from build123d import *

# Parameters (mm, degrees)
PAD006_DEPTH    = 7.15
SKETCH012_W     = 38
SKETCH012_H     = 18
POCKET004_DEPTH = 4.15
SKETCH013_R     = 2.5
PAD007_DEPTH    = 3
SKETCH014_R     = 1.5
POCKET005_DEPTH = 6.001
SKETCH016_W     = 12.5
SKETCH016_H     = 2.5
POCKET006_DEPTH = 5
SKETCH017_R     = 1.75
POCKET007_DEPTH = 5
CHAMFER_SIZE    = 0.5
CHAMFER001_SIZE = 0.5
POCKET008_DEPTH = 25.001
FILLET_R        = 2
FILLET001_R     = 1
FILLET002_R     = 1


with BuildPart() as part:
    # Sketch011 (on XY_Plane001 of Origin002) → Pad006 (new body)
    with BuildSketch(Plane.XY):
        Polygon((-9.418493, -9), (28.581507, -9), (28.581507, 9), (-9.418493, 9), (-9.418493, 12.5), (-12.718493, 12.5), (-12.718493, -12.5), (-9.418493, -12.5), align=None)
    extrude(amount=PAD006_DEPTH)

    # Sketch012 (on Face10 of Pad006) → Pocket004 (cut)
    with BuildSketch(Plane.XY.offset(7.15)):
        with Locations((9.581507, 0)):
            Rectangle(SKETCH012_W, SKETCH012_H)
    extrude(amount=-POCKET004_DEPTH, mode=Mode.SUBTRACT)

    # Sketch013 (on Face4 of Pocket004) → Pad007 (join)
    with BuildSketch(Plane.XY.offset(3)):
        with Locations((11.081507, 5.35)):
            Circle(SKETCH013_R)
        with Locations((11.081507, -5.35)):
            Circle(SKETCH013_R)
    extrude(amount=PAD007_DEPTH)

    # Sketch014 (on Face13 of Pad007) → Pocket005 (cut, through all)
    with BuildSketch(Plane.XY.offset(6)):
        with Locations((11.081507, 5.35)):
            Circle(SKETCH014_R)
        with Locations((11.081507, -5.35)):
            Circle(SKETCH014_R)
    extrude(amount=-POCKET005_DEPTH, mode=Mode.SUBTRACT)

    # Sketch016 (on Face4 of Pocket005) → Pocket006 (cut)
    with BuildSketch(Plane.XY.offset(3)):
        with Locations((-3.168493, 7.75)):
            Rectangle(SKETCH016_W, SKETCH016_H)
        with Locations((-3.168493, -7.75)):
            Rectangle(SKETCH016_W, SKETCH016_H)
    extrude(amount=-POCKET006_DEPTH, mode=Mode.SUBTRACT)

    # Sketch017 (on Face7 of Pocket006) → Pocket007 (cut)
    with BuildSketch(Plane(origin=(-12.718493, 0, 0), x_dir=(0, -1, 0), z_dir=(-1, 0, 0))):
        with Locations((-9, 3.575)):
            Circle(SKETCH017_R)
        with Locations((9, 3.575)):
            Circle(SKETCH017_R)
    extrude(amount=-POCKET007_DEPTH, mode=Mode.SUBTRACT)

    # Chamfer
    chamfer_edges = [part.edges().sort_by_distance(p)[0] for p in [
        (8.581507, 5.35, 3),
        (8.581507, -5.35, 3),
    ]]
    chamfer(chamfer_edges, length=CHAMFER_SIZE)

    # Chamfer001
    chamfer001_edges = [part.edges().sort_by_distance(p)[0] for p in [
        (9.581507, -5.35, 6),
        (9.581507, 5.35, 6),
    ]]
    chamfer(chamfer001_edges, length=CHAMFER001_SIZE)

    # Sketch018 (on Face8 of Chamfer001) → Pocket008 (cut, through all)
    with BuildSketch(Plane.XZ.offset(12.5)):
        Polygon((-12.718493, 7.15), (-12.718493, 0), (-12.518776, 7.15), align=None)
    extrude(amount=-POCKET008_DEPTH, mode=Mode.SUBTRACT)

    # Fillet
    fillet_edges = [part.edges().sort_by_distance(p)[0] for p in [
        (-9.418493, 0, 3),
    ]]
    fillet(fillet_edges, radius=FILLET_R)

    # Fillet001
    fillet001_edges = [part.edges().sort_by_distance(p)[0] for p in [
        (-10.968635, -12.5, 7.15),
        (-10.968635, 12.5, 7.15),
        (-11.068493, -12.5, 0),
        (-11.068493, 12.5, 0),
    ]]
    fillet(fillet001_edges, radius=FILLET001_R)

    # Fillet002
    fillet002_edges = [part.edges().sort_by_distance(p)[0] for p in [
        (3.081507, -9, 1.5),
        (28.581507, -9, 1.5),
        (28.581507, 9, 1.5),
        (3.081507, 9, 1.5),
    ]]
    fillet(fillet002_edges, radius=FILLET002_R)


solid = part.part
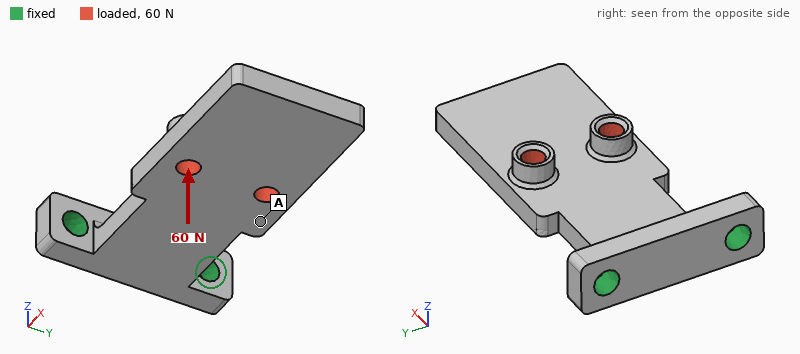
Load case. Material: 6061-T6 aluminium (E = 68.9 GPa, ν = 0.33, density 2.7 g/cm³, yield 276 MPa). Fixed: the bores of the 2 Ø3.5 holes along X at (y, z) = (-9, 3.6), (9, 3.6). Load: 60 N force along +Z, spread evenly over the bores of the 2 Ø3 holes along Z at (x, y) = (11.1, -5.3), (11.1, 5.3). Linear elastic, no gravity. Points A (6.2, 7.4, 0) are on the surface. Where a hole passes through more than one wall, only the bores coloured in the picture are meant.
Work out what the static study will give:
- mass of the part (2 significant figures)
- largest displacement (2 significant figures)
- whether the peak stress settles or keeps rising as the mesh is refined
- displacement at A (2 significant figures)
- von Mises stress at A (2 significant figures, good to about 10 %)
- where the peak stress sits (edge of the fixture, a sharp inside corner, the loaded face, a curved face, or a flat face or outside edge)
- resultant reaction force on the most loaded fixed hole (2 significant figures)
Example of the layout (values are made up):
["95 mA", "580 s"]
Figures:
["6.5 g", "0.24 mm", "keeps rising", "0.078 mm", "8.9 MPa", "a sharp inside corner", "31 N"]
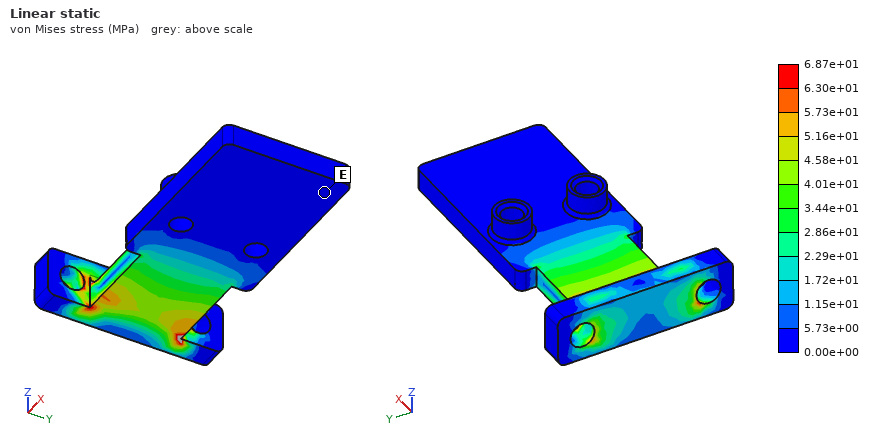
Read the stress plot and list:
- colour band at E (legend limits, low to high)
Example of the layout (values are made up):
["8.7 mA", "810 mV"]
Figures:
["0.00e+00 to 5.73e+00 MPa"]
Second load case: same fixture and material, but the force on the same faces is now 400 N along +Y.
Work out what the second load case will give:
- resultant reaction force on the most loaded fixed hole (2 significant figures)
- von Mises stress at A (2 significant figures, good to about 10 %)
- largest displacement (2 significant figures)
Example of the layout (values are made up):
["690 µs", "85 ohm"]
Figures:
["670 N", "11 MPa", "0.13 mm"]
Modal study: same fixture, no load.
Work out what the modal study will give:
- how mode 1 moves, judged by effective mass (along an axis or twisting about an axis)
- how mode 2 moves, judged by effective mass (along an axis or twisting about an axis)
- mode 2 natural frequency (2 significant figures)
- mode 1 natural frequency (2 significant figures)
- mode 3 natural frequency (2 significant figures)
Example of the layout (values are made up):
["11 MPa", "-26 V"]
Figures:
["along Z", "along Y", "4800 Hz", "1300 Hz", "6000 Hz"]
